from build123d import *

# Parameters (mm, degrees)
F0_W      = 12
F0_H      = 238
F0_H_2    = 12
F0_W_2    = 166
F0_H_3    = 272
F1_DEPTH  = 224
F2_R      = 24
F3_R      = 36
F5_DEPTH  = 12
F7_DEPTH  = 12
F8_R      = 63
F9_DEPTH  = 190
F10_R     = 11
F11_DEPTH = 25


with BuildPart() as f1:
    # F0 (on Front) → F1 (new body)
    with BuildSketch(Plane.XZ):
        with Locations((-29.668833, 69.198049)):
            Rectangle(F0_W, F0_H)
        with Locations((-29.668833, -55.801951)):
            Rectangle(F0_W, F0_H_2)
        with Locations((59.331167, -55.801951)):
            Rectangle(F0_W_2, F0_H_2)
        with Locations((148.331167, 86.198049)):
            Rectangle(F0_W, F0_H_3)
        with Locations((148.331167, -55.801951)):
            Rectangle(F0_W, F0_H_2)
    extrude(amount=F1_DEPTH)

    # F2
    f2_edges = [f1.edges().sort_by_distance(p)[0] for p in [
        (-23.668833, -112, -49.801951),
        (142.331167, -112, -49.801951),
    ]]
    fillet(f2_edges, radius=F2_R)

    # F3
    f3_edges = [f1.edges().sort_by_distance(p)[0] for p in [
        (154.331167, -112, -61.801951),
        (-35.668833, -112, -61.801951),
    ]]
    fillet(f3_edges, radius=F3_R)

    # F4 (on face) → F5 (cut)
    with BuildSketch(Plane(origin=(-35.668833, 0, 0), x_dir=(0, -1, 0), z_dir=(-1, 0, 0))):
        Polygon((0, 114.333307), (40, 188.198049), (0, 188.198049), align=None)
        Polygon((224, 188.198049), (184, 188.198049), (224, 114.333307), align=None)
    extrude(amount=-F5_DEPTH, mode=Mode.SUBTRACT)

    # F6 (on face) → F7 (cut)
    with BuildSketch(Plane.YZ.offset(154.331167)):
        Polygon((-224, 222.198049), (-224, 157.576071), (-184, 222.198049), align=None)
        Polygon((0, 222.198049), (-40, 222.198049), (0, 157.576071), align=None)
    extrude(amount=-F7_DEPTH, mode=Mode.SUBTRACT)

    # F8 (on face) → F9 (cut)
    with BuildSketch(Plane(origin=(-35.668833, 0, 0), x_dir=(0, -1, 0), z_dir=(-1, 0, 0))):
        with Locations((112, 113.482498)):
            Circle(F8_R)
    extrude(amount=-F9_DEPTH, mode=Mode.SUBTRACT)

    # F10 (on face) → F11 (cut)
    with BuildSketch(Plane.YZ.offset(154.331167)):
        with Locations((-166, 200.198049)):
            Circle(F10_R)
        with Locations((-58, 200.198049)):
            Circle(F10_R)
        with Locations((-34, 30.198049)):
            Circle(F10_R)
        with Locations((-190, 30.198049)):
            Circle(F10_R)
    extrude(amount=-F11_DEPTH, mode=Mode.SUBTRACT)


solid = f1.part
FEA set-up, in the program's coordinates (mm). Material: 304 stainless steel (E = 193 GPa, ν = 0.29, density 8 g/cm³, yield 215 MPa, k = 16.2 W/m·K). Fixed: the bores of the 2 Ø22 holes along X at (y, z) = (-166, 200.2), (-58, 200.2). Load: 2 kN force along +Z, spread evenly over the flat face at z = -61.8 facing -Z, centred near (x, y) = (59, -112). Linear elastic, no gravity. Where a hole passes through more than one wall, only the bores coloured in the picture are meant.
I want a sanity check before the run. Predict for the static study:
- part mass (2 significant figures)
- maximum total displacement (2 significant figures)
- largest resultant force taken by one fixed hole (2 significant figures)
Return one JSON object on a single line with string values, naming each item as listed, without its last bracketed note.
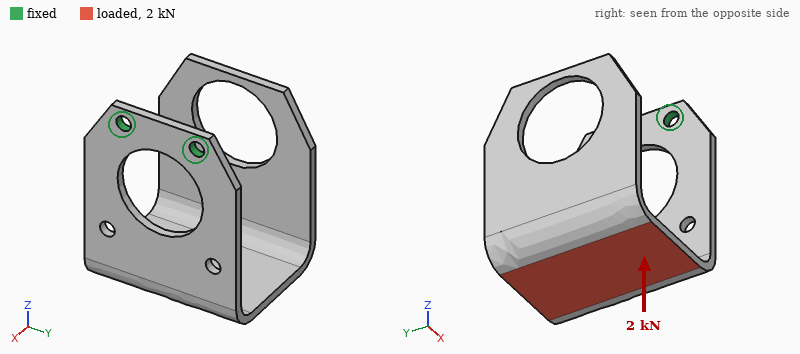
{"part mass": "11 kg", "maximum total displacement": "2.7 mm", "largest resultant force taken by one fixed hole": "1.0 kN"}
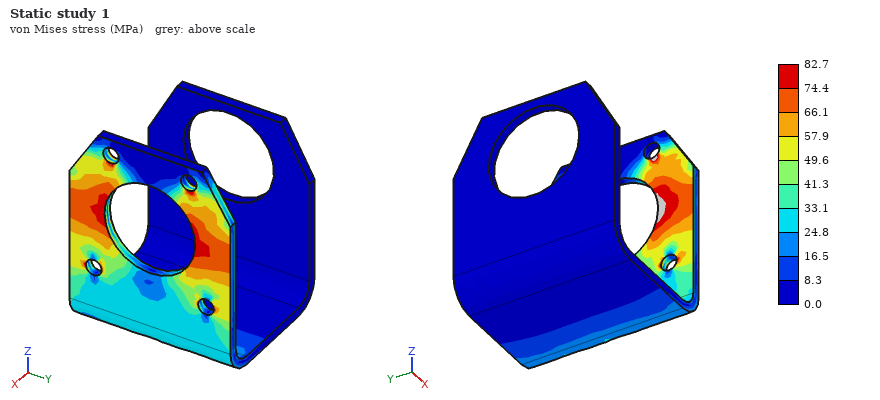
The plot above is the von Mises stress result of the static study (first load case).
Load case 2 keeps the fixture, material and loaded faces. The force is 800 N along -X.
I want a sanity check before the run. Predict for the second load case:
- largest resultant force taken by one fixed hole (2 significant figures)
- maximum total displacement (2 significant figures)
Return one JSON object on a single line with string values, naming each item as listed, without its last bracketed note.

{"largest resultant force taken by one fixed hole": "400 N", "maximum total displacement": "1.9 mm"}
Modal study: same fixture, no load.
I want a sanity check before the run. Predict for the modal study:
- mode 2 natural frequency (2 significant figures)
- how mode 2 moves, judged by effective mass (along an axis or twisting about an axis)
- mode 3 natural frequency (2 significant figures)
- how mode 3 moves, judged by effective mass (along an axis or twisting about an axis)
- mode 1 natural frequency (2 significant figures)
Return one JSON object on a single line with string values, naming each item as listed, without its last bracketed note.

{"mode 2 natural frequency": "63 Hz", "how mode 2 moves, judged by effective mass": "along Y", "mode 3 natural frequency": "84 Hz", "how mode 3 moves, judged by effective mass": "along X", "mode 1 natural frequency": "37 Hz"}
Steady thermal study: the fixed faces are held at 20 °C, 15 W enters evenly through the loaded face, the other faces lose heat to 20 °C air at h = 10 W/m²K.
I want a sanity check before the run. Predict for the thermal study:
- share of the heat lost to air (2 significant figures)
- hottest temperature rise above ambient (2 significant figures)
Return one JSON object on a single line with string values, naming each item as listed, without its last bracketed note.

{"share of the heat lost to air": "98 %", "hottest temperature rise above ambient": "16 K"}
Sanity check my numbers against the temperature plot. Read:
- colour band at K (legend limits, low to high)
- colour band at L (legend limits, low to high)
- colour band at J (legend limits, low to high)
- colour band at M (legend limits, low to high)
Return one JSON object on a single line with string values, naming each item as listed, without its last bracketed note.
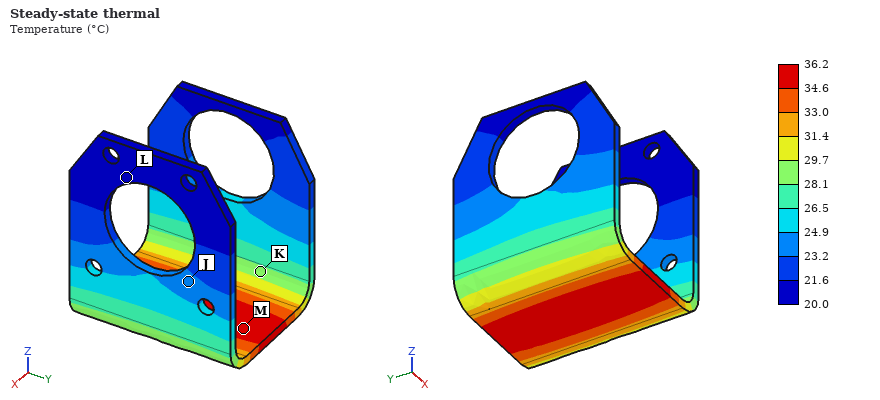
{"colour band at K": "28.1 to 29.7 °C", "colour band at L": "20.0 to 21.6 °C", "colour band at J": "23.2 to 24.9 °C", "colour band at M": "34.6 to 36.2 °C"}
